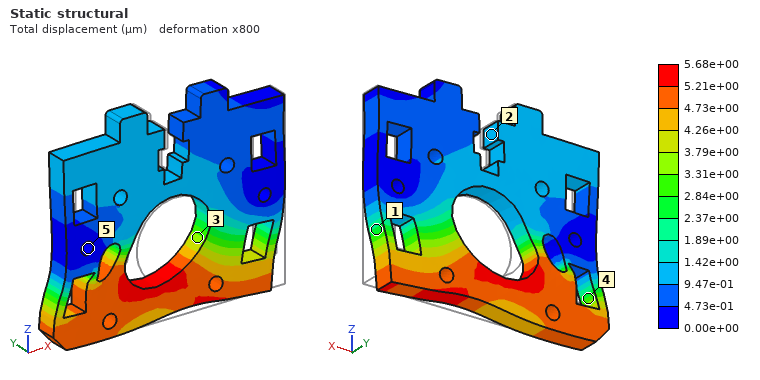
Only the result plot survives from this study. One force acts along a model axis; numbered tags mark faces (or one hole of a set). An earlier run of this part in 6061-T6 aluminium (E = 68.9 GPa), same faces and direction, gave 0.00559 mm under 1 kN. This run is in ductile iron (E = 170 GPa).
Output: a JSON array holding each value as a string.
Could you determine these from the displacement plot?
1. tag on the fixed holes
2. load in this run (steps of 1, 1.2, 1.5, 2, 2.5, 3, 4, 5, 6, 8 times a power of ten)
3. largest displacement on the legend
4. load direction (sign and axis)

["5", "2.5 kN", "5.68e+00 µm", "-X"]
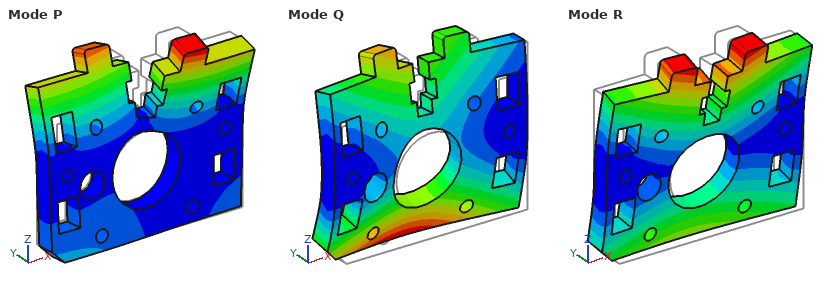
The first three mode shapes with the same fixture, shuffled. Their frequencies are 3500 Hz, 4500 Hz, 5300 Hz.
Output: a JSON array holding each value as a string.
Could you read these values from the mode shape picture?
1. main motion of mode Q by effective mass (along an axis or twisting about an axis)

["along Y"]
